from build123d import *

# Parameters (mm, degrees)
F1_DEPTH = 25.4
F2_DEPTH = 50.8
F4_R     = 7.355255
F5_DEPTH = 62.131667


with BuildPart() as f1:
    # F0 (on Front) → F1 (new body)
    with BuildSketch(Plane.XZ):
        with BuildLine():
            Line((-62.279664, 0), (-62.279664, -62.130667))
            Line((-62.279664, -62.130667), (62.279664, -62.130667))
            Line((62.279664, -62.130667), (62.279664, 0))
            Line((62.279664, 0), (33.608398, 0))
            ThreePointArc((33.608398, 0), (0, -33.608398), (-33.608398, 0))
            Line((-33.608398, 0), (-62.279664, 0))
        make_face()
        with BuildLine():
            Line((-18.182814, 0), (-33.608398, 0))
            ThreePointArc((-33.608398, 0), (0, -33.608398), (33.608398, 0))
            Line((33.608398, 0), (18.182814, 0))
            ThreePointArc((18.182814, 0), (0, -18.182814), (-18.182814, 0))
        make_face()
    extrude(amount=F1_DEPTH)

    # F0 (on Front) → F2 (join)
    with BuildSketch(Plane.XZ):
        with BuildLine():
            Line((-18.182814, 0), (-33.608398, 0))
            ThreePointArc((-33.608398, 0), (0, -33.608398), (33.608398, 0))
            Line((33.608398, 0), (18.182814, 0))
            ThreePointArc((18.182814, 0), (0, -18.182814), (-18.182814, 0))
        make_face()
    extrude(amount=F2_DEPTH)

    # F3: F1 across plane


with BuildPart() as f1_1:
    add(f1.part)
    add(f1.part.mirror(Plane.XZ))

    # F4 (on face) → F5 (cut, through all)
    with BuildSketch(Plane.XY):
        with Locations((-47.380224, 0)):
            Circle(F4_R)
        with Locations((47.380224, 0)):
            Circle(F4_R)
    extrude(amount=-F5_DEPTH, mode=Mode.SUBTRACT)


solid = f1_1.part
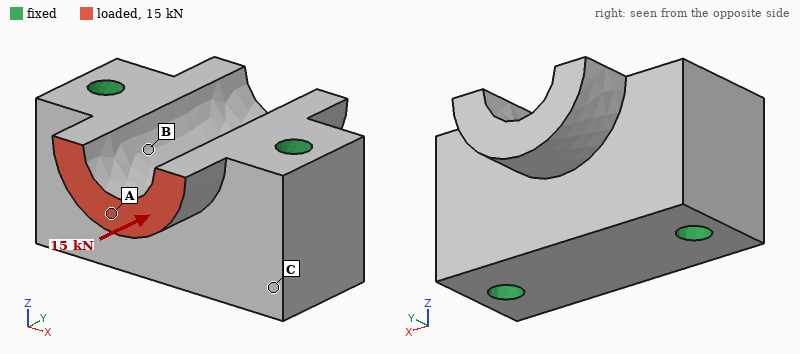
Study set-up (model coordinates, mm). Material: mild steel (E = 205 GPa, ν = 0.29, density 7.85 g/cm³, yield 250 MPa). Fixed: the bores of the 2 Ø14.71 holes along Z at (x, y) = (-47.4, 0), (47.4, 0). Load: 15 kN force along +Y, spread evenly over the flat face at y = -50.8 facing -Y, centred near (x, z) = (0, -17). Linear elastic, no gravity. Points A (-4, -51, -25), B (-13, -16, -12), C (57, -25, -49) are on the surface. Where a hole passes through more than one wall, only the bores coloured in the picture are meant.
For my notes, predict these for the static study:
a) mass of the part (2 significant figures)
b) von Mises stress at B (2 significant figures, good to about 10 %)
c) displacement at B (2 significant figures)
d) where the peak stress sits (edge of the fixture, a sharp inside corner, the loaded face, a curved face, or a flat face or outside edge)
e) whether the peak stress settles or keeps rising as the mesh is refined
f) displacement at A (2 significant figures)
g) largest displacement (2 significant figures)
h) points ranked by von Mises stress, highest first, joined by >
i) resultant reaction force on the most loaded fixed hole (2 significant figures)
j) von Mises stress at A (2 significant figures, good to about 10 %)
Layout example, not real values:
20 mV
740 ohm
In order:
3.2 kg
6.4 MPa
2.1 µm
edge of the fixture
keeps rising
3.3 µm
4.5 µm
A > B > C
7.6 kN
11 MPa
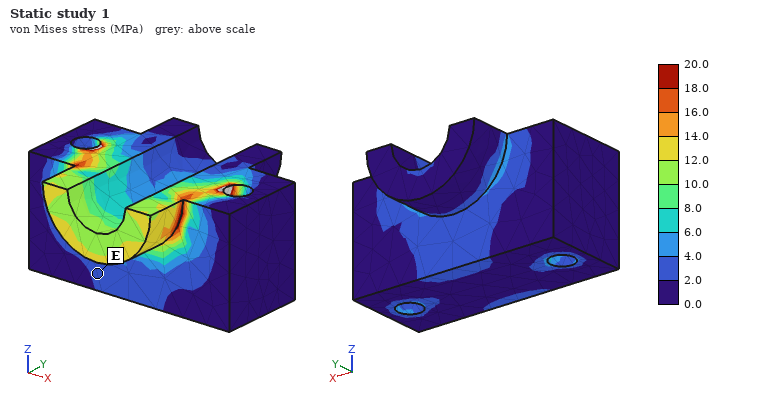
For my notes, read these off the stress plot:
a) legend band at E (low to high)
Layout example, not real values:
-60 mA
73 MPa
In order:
2.0 to 4.0 MPa
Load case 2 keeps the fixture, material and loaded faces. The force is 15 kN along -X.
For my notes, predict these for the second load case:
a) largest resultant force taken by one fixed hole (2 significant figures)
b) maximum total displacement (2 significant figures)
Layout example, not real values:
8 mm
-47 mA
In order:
11 kN
22 µm
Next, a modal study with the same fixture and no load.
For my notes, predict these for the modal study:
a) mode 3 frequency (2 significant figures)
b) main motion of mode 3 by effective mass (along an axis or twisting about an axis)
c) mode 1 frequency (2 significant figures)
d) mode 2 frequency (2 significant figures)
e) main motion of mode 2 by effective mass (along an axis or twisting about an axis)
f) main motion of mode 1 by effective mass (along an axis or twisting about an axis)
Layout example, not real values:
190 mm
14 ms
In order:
12 kHz
along Y
10 kHz
11 kHz
along Z
twisting about X
